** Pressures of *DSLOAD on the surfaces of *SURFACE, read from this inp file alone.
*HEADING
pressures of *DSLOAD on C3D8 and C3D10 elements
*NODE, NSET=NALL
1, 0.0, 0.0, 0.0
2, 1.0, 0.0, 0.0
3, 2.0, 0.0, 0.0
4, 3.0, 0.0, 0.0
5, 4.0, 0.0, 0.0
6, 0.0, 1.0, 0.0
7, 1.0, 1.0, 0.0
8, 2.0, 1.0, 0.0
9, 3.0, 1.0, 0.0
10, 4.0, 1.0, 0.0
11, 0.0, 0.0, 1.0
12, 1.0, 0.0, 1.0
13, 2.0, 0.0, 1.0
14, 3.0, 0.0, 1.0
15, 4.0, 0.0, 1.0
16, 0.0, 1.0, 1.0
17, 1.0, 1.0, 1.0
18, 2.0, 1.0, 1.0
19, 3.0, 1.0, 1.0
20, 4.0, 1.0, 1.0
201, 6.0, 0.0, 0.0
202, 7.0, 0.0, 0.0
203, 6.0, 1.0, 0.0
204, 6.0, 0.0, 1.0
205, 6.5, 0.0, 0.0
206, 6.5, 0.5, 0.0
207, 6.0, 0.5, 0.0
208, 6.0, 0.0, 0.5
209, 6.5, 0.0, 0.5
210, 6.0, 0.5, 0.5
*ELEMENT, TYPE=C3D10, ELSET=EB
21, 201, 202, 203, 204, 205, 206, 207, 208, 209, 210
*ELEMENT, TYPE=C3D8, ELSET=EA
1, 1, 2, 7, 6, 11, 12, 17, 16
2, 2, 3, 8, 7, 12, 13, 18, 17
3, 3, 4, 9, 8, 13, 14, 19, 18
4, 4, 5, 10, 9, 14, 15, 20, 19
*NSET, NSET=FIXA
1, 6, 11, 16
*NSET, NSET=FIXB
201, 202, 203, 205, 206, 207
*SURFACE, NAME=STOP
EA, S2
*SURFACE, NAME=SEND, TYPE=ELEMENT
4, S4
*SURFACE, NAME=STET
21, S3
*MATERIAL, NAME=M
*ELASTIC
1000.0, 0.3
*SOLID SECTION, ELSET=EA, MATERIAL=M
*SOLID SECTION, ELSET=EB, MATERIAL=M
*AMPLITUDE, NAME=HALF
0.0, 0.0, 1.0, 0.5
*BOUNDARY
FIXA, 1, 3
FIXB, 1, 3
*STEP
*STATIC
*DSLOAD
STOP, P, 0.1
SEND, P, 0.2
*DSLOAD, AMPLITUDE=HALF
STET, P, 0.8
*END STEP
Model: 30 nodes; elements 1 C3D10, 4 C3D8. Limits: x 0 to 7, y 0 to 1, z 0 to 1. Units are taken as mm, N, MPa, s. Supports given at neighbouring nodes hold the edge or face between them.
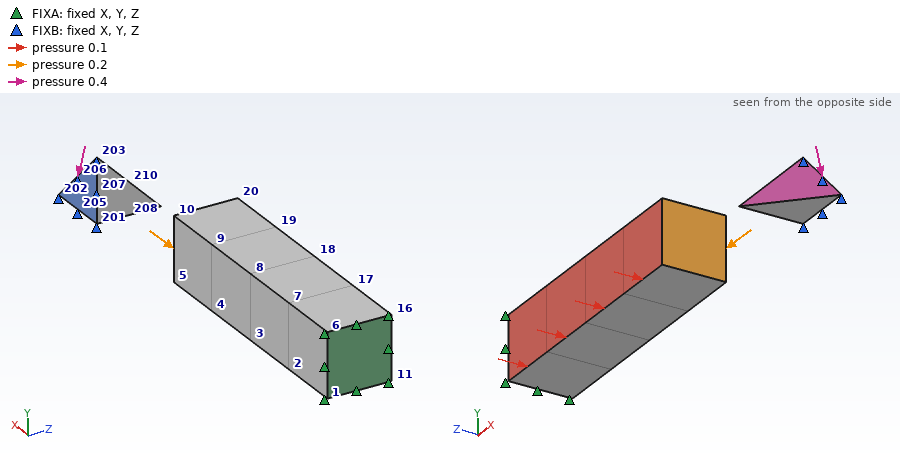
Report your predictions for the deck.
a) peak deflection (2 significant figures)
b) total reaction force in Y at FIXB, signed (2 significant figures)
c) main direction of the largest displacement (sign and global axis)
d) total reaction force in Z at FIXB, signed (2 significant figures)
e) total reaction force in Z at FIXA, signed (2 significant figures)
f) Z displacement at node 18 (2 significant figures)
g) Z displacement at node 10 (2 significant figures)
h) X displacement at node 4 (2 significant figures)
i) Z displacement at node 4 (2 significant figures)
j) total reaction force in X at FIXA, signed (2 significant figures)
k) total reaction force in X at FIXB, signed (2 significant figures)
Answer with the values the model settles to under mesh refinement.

0.039 mm
0.20 N
-Z
0.20 N
0.40 N
-0.014 mm
-0.038 mm
-0.0066 mm
-0.026 mm
0.20 N
0.20 N
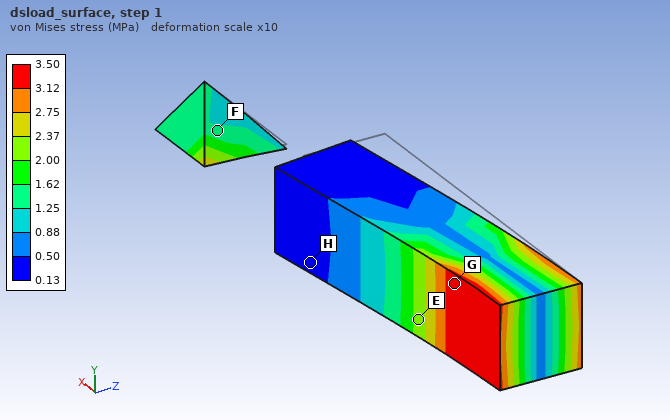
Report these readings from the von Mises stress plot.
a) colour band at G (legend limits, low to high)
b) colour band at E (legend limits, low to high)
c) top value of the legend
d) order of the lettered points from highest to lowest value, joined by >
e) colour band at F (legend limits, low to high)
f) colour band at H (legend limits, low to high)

3.12 to 3.50 MPa
2.00 to 2.37 MPa
3.50 MPa
G > E > F > H
1.25 to 1.62 MPa
0.13 to 0.50 MPa
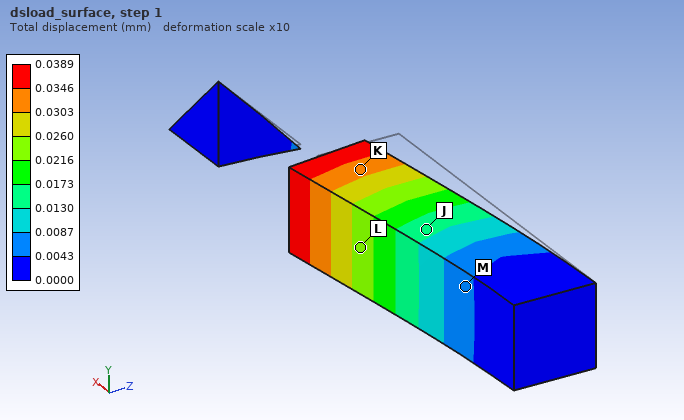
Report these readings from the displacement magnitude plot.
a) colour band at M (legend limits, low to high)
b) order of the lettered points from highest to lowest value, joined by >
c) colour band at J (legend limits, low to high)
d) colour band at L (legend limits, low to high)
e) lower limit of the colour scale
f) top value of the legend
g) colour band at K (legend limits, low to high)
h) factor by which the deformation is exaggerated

0.0043 to 0.0087 mm
K > L > J > M
0.0130 to 0.0173 mm
0.0216 to 0.0260 mm
0.0000 mm
0.0389 mm
0.0303 to 0.0346 mm
10
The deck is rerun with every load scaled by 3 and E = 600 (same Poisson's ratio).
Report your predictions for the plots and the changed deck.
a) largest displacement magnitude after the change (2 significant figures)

0.19 mm
